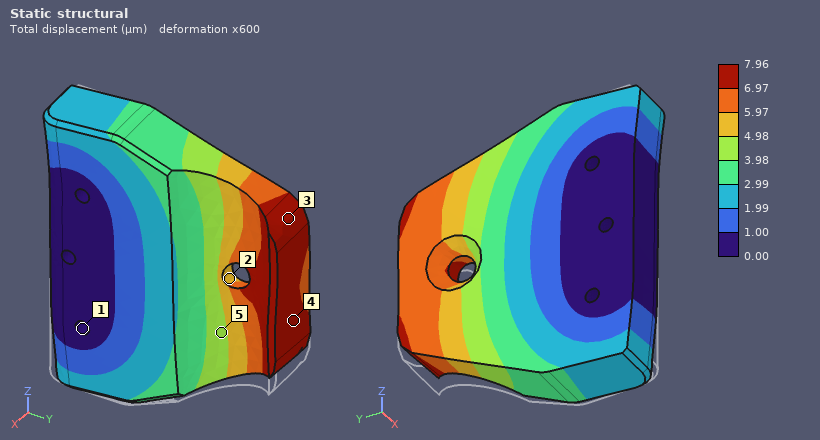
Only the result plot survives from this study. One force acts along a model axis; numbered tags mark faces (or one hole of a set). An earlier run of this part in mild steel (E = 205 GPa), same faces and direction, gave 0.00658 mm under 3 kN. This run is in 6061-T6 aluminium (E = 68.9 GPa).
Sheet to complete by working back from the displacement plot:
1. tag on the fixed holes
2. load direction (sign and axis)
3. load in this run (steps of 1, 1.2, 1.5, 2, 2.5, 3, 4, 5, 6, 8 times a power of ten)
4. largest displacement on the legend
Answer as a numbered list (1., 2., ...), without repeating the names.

1. 1
2. +Z
3. 1.2 kN
4. 7.96 µm
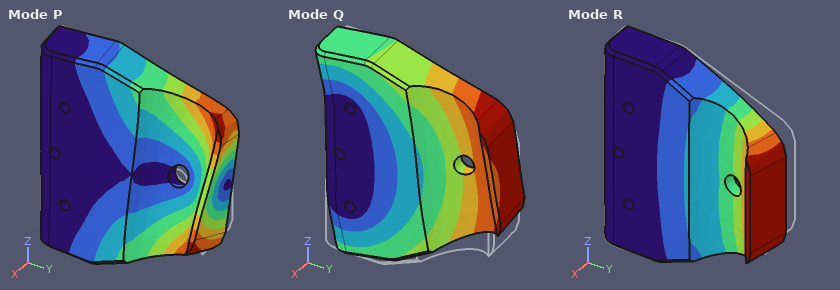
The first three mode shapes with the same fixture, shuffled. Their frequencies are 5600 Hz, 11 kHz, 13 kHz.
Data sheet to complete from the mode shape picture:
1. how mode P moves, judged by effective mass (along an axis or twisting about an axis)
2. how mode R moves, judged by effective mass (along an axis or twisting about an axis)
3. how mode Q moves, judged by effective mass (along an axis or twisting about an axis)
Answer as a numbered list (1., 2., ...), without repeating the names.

1. twisting about Y
2. along X
3. along Z
